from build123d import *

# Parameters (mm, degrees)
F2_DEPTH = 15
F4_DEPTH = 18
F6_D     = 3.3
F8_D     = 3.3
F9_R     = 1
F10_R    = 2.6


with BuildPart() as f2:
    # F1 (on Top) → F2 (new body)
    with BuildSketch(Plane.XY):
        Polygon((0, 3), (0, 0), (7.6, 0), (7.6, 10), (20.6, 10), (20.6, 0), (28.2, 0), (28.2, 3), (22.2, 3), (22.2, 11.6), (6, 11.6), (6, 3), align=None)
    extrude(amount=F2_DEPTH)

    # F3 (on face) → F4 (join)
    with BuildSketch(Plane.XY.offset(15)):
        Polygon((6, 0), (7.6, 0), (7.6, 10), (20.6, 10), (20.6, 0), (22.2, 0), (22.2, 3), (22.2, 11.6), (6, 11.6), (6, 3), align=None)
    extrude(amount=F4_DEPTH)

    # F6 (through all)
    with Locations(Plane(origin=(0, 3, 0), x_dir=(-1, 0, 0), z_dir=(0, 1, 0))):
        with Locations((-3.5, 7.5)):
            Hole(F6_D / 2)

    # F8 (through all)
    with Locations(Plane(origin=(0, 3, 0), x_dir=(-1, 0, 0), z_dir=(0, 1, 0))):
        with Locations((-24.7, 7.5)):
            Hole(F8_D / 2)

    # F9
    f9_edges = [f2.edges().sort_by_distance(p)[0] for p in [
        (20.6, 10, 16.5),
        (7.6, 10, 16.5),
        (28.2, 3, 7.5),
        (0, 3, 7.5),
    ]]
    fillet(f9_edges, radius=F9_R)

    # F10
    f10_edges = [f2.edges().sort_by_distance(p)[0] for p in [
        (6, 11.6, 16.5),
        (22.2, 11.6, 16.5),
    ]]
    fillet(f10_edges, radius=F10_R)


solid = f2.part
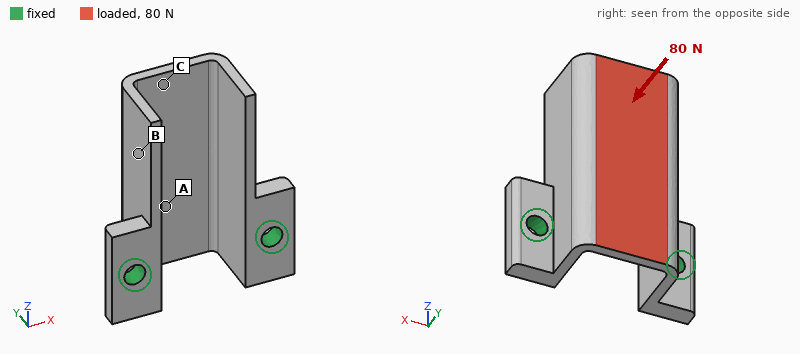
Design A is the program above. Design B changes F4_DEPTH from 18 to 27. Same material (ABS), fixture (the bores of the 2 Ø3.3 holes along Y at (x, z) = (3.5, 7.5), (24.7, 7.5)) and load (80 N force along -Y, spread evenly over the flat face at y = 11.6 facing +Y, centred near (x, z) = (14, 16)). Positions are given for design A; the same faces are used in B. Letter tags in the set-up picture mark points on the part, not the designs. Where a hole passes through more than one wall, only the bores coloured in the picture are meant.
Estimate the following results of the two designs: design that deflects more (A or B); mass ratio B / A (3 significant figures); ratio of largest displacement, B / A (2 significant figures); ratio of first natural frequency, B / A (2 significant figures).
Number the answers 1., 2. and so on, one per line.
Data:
1. B
2. 1.22
3. 1.9
4. 0.63
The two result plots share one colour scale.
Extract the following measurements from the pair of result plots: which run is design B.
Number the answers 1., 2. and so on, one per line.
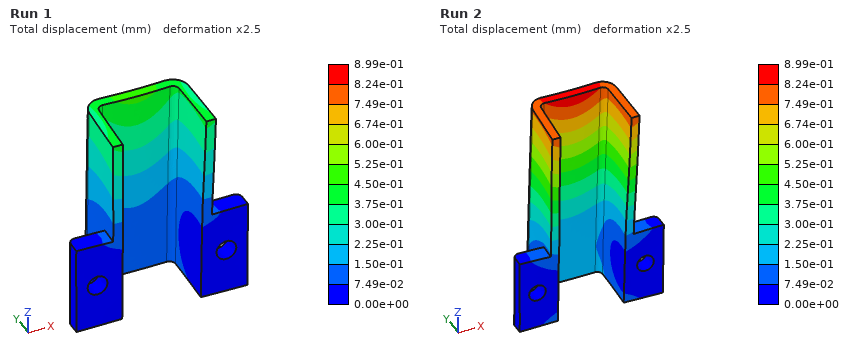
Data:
1. Run 2
